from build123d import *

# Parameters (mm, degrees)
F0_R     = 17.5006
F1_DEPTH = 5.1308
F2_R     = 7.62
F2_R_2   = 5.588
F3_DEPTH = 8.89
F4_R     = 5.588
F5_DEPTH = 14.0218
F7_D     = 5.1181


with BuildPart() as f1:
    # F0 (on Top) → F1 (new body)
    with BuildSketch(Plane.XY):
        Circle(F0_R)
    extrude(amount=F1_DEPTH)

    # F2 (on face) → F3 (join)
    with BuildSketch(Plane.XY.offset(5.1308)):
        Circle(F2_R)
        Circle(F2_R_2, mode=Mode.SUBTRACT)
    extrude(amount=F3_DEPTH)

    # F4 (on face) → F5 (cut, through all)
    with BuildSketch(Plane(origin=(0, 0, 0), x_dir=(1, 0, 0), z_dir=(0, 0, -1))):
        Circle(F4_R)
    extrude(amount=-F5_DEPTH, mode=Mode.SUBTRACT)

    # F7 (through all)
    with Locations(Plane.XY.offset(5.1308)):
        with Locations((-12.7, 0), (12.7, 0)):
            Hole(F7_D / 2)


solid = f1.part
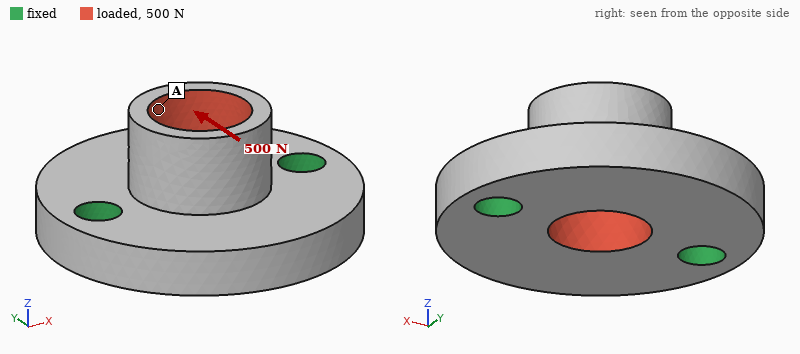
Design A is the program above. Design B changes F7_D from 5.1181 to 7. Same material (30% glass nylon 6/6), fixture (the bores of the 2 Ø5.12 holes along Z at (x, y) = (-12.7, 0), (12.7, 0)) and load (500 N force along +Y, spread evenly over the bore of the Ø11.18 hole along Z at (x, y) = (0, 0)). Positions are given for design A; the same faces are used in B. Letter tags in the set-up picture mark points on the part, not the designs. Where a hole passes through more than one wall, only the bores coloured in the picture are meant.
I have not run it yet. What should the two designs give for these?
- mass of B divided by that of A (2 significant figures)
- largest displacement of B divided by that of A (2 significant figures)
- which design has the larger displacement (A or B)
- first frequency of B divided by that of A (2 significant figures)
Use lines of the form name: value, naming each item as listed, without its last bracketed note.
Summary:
mass of B divided by that of A: 0.96
largest displacement of B divided by that of A: 0.81
which design has the larger displacement: A
first frequency of B divided by that of A: 1.2
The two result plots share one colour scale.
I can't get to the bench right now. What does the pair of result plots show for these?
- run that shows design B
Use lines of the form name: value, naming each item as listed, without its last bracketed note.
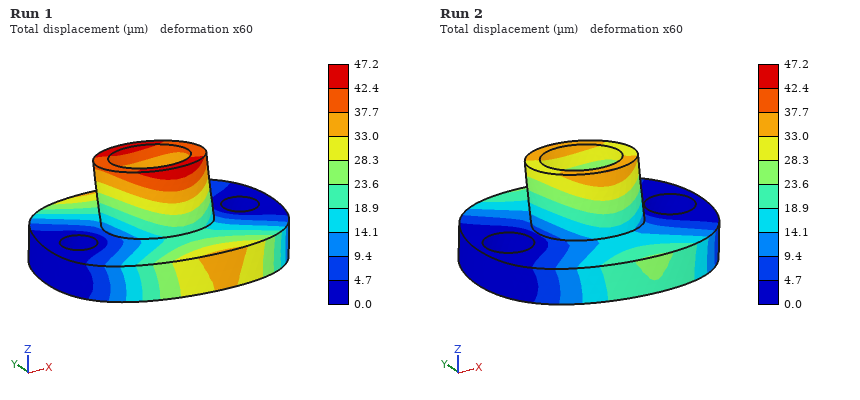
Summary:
run that shows design B: Run 2
